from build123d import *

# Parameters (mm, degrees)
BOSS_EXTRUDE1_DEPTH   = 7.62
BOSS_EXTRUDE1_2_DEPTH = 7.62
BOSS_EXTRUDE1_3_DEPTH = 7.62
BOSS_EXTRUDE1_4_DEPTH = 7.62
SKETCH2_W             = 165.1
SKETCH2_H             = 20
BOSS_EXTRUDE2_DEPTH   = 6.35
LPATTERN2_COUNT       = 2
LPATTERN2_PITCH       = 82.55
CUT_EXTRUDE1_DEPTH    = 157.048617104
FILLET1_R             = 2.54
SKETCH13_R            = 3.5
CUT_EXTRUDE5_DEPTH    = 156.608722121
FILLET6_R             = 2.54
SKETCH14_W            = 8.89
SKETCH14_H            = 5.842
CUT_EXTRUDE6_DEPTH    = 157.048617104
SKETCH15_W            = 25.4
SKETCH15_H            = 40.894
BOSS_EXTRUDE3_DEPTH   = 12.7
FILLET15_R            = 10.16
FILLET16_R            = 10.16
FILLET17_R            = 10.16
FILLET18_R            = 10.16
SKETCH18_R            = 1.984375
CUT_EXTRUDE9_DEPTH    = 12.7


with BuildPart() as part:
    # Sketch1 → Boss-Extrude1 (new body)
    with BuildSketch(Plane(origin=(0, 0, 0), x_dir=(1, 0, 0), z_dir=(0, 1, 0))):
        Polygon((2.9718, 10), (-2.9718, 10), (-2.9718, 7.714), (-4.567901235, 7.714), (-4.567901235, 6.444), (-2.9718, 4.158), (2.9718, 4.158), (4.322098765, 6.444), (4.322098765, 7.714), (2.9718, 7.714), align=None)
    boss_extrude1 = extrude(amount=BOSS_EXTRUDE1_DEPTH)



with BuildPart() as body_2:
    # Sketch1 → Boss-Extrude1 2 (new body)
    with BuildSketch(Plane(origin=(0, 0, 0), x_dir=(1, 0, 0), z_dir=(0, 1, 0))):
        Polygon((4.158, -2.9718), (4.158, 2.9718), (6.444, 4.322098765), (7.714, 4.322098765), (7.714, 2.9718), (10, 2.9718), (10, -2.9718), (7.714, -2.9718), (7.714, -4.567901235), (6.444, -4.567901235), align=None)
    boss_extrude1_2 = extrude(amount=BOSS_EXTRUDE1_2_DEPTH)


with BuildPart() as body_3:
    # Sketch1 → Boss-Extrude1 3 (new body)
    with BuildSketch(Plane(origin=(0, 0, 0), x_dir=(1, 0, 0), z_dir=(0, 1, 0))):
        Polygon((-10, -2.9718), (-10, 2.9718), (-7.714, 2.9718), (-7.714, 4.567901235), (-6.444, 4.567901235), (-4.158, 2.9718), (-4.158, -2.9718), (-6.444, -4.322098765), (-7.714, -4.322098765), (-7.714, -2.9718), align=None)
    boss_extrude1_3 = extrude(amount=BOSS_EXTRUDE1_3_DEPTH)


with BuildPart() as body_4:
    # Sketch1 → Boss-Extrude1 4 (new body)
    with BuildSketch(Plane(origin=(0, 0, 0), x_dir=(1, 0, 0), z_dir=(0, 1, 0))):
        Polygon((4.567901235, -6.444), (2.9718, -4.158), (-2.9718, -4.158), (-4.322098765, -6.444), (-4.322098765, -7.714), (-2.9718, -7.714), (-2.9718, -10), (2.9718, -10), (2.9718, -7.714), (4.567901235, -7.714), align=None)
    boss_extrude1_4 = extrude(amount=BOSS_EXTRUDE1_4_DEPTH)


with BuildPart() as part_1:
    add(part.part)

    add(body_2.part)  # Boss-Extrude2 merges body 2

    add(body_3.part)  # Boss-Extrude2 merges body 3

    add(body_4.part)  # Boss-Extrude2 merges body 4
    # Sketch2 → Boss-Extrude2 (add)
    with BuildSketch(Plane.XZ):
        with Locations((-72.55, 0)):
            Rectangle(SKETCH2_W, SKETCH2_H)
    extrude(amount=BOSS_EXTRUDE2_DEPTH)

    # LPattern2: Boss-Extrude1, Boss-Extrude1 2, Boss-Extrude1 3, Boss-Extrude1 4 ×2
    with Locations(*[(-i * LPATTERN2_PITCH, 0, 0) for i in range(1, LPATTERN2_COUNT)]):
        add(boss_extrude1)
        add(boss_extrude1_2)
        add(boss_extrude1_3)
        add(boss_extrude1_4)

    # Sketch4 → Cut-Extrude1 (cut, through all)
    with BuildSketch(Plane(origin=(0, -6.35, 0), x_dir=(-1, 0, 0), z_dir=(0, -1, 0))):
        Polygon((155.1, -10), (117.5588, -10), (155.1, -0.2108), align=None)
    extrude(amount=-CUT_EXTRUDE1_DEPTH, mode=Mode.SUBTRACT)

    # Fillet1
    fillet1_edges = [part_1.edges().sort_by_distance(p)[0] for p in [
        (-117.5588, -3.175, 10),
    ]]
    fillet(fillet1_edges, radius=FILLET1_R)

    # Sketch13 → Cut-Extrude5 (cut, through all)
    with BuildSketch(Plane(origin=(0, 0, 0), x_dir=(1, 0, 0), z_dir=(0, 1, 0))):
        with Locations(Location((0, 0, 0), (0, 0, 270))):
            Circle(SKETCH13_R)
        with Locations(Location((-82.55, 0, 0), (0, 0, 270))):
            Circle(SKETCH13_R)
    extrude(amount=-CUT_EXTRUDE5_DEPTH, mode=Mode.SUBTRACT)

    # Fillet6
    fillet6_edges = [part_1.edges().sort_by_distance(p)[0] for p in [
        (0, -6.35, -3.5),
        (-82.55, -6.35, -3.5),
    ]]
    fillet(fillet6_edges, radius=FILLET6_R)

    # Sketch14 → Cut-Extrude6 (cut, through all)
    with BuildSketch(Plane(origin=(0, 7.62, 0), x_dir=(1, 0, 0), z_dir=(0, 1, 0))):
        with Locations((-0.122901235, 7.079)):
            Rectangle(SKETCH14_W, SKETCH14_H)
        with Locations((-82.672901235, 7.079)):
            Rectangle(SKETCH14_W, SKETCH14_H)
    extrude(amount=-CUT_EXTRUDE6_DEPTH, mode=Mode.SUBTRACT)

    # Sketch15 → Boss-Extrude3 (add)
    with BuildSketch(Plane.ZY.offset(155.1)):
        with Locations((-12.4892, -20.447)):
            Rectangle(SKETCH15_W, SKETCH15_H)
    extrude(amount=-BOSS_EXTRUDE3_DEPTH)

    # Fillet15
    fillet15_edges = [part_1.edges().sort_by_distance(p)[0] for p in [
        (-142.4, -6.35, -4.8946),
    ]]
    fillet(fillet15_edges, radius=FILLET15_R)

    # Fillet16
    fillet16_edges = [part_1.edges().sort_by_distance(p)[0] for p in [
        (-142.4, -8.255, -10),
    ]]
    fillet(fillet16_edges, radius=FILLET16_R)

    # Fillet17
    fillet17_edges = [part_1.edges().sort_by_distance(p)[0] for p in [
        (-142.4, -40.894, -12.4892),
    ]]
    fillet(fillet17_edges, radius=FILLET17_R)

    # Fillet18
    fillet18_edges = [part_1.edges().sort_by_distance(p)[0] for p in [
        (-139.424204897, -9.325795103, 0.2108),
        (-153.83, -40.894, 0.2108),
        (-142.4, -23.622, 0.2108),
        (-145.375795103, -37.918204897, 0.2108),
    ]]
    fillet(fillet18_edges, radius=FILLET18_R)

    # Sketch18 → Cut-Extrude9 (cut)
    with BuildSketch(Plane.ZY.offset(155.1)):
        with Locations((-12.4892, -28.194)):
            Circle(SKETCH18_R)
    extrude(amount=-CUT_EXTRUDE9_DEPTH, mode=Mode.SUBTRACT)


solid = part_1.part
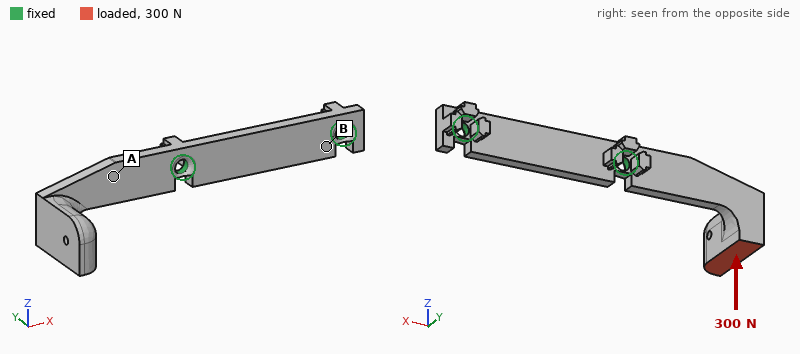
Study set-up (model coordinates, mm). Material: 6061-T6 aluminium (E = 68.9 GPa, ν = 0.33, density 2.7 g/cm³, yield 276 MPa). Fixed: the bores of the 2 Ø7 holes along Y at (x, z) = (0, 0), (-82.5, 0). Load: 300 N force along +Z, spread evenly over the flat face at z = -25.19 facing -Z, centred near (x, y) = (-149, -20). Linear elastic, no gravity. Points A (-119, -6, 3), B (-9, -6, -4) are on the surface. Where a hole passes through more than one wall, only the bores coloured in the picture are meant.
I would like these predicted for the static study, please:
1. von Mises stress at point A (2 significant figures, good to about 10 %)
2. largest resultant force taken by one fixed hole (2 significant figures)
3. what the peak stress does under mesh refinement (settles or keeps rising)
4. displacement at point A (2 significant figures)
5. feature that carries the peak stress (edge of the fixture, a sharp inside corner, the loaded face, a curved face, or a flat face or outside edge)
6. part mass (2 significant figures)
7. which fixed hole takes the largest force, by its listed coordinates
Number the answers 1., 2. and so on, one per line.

1. 43 MPa
2. 390 N
3. keeps rising
4. 0.11 mm
5. edge of the fixture
6. 86 g
7. (-82.5, 0)
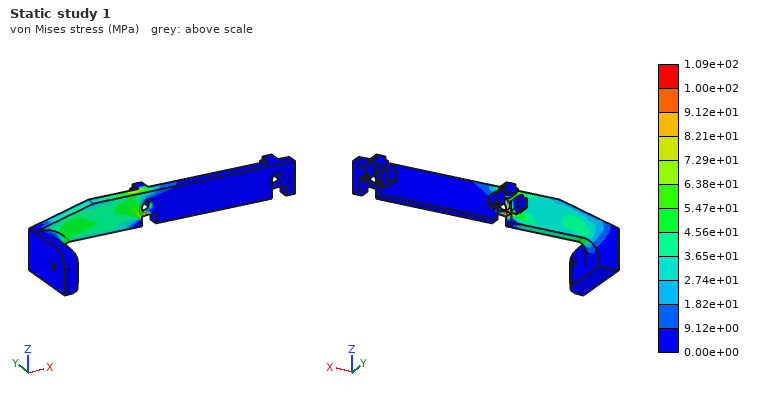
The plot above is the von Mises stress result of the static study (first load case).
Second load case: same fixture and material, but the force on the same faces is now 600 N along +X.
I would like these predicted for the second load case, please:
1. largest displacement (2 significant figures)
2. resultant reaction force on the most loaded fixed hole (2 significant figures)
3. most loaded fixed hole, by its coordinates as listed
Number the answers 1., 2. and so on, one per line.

1. 1.5 mm
2. 650 N
3. (-82.5, 0)
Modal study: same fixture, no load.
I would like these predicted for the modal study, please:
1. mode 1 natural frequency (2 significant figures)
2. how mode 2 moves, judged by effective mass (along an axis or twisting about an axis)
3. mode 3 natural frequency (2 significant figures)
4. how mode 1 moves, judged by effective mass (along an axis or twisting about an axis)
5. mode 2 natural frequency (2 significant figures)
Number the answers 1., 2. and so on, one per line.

1. 390 Hz
2. along Z
3. 1800 Hz
4. along Y
5. 740 Hz
